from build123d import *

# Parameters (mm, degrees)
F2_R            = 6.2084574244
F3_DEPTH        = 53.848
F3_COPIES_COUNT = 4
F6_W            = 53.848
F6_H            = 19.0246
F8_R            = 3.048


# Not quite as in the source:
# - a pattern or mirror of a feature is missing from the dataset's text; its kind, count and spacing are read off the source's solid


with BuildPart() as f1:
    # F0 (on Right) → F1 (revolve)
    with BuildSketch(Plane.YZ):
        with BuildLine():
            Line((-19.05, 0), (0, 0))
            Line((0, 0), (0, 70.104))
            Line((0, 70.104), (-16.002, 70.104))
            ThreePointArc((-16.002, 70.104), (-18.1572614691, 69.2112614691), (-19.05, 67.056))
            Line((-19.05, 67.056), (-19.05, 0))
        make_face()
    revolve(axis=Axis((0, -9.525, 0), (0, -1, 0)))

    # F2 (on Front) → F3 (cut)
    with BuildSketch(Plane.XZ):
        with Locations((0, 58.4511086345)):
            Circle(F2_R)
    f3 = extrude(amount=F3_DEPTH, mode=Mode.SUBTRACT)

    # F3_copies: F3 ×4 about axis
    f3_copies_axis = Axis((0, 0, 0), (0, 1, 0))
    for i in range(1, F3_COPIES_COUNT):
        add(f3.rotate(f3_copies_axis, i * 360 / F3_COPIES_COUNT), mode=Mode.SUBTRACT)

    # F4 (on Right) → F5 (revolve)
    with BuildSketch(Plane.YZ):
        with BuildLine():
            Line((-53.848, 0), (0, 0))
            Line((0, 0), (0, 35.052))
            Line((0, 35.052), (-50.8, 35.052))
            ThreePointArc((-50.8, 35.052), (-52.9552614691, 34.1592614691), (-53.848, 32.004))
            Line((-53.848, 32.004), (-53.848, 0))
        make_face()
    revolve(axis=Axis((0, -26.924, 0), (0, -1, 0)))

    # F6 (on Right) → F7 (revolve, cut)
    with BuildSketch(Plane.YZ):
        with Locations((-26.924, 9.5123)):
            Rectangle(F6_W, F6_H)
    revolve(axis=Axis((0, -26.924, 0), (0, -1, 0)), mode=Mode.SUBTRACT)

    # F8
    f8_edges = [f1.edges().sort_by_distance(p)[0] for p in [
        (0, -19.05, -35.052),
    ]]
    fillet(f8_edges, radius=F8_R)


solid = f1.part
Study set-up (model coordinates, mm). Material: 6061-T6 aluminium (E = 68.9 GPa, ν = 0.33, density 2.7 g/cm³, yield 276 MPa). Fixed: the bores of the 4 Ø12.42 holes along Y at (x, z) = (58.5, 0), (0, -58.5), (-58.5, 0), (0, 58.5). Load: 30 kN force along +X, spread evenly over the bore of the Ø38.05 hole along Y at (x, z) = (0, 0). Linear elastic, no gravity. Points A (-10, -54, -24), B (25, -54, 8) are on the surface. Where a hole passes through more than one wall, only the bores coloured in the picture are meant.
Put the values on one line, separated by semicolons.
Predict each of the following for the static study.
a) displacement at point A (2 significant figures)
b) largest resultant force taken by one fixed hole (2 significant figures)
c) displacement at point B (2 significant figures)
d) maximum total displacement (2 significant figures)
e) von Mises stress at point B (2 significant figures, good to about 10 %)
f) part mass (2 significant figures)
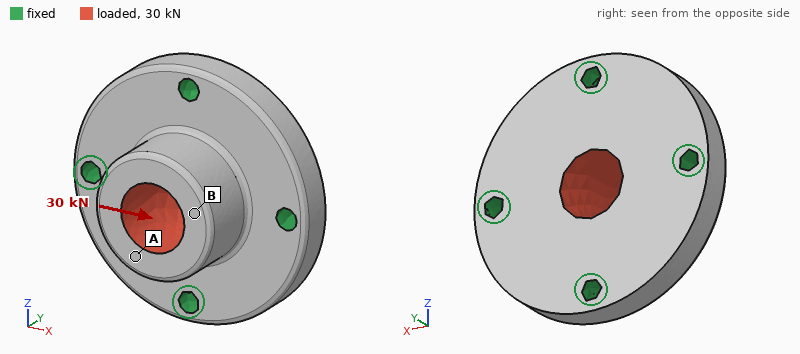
24 µm; 11 kN; 28 µm; 28 µm; 9.7 MPa; 960 g
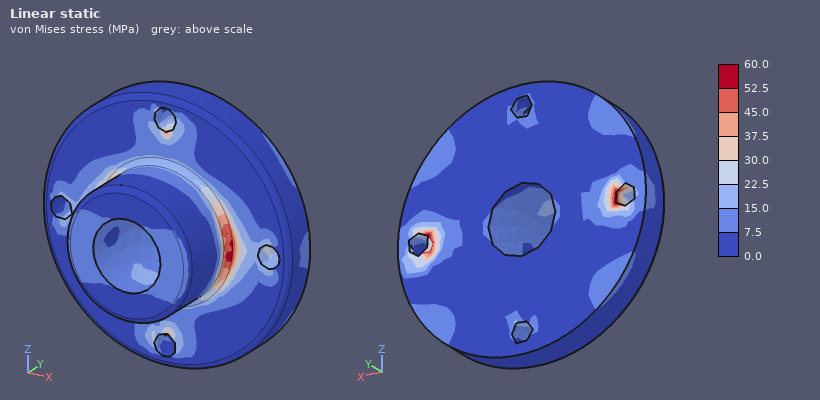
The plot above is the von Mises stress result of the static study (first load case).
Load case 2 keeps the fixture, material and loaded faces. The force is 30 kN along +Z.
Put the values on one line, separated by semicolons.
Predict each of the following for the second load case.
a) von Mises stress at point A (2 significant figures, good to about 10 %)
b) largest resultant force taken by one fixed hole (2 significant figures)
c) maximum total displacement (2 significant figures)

9.5 MPa; 11 kN; 28 µm
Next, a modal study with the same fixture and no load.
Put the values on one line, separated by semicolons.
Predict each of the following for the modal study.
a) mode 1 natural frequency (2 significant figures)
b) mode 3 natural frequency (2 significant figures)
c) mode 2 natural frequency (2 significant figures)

8200 Hz; 8500 Hz; 8500 Hz
